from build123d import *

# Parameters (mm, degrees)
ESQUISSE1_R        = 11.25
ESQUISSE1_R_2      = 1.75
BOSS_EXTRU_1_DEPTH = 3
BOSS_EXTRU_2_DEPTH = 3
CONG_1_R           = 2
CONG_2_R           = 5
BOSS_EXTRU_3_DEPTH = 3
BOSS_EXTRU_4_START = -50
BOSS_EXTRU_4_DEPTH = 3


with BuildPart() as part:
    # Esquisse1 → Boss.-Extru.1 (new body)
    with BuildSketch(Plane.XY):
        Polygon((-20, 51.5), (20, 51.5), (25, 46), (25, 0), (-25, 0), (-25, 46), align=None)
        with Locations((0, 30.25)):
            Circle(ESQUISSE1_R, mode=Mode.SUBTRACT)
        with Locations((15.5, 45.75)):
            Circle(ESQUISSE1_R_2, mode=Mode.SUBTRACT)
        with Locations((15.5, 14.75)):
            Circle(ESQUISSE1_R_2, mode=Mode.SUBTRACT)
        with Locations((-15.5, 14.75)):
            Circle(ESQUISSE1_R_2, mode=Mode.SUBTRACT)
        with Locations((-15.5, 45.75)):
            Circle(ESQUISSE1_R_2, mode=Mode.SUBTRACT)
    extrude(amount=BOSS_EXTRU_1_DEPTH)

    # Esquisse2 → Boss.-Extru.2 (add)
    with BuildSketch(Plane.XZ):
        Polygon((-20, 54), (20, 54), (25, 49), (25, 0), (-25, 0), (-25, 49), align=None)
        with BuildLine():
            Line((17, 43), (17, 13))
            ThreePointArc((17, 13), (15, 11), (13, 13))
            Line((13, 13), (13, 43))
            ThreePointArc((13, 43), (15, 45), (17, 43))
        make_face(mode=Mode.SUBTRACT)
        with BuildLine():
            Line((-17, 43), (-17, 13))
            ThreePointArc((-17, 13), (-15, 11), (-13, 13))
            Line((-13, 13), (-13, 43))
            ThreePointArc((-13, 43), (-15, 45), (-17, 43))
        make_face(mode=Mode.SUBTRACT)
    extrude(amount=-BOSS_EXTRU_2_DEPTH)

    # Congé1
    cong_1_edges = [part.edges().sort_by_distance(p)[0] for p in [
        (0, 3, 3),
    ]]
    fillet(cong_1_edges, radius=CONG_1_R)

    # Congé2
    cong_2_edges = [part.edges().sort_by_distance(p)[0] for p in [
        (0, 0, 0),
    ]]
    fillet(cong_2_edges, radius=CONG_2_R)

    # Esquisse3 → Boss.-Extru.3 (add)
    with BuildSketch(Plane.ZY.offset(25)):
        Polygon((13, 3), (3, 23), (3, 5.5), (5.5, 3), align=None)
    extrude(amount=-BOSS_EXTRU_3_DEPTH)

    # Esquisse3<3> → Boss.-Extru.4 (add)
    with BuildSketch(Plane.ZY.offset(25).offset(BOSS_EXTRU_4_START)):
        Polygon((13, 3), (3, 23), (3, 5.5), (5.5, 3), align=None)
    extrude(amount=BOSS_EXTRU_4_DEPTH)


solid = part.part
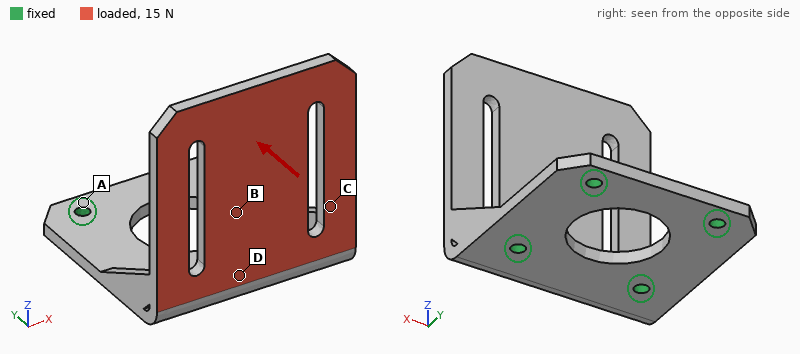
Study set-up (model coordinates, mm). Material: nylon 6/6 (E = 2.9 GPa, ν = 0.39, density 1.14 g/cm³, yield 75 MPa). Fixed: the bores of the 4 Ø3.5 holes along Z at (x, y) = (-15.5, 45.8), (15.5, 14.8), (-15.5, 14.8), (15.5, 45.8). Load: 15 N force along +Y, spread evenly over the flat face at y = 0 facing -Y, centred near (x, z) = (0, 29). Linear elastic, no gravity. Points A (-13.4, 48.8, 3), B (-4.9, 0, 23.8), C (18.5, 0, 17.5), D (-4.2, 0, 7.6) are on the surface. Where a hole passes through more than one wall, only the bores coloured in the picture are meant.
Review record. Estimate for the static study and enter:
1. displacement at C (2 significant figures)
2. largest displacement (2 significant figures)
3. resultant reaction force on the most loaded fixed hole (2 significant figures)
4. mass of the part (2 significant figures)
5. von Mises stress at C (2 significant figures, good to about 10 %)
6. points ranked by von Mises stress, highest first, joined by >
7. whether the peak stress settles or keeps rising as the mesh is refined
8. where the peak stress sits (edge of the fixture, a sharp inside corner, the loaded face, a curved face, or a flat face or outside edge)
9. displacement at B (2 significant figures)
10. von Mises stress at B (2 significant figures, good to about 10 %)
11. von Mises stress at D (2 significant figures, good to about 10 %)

0.17 mm
1.1 mm
8.7 N
15 g
4.4 MPa
C > D > B > A
keeps rising
edge of the fixture
0.34 mm
1.7 MPa
2.7 MPa
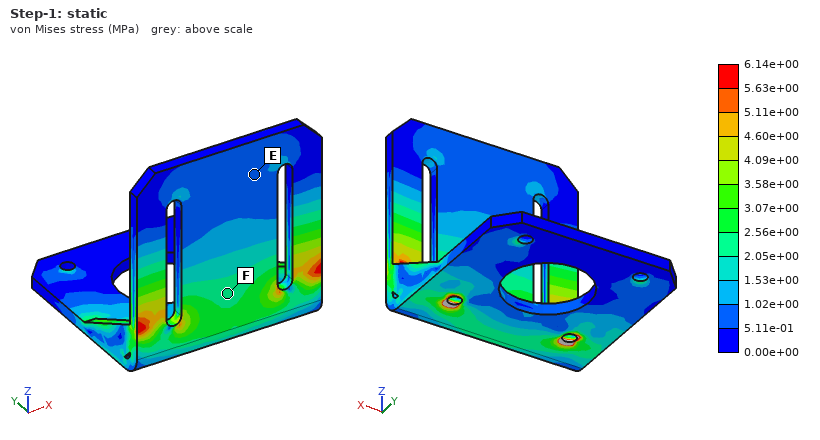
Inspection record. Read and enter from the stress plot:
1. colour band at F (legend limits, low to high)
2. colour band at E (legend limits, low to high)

2.05e+00 to 2.56e+00 MPa
5.11e-01 to 1.02e+00 MPa
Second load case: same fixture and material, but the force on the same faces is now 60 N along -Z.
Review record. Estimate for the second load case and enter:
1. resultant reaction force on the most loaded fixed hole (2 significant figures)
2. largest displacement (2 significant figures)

35 N
0.82 mm
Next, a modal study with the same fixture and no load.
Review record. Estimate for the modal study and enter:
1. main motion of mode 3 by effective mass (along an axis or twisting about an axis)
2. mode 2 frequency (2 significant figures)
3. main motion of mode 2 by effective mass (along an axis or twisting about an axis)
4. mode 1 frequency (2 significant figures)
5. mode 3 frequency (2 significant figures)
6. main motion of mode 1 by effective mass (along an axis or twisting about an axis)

along X
640 Hz
along X
270 Hz
940 Hz
along Y
